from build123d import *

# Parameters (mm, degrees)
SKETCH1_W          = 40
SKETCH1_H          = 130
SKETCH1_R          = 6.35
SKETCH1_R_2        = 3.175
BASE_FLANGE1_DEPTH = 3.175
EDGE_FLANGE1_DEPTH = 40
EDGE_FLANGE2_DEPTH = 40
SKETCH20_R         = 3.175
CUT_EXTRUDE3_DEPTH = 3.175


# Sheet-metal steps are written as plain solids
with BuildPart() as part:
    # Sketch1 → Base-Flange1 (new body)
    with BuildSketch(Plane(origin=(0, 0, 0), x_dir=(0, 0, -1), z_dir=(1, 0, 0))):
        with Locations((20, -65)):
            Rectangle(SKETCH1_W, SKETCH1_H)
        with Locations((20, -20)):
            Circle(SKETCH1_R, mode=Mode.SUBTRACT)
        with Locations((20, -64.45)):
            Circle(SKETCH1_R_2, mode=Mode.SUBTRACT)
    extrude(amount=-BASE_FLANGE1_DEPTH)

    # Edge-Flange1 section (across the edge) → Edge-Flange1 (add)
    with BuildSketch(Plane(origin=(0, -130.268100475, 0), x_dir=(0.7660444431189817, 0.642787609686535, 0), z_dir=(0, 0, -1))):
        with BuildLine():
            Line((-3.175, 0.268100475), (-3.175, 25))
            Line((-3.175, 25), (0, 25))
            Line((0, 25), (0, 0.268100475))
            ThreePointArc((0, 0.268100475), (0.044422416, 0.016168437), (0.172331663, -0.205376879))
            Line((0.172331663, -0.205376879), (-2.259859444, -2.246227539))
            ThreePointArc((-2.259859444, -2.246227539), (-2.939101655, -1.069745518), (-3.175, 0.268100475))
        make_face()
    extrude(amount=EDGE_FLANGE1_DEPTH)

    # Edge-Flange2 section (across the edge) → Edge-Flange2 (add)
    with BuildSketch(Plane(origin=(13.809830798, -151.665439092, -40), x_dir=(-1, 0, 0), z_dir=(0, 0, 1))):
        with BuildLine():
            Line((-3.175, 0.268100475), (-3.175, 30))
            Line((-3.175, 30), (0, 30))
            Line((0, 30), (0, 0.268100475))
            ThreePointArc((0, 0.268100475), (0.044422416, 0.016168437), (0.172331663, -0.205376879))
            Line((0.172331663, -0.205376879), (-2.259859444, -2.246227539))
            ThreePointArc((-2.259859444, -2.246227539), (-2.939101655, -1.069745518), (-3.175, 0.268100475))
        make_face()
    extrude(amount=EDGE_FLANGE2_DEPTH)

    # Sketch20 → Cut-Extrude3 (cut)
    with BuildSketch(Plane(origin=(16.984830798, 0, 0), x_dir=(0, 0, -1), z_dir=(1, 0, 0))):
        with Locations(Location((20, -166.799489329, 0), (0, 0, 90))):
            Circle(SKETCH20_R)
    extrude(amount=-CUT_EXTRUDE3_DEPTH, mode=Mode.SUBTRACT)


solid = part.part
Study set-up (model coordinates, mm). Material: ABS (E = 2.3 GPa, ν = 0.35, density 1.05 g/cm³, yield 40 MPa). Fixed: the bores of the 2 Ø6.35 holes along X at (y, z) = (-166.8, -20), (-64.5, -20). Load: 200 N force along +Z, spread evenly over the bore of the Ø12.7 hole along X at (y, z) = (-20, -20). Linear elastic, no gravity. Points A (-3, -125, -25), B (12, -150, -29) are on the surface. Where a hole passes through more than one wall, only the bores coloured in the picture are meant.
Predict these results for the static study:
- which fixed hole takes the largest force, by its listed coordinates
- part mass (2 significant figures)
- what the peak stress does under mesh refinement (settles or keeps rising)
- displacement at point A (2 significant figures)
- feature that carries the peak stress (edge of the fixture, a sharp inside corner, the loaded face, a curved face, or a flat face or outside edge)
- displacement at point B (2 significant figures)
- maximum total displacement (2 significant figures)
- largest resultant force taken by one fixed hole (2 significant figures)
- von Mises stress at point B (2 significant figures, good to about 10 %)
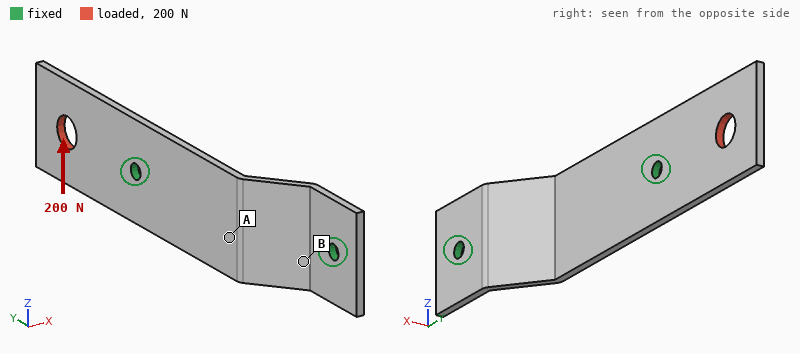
(-64.5, -20)
24 g
keeps rising
0.62 mm
edge of the fixture
0.29 mm
1.2 mm
250 N
5.6 MPa
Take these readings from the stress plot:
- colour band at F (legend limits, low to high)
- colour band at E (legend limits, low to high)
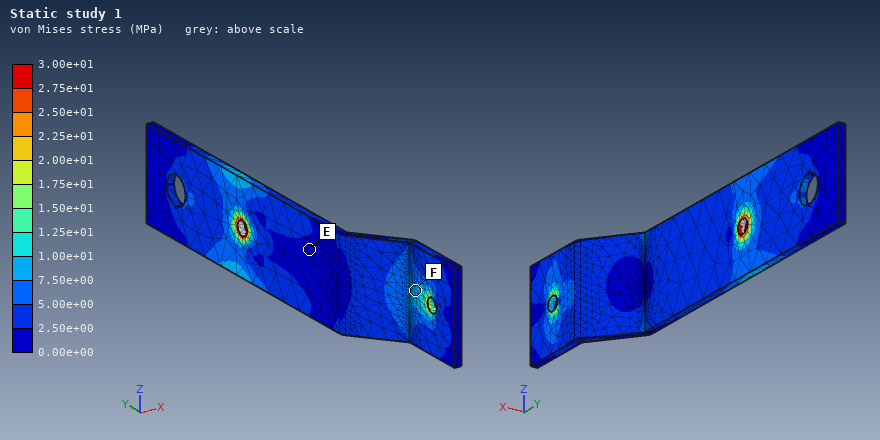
7.50e+00 to 1.00e+01 MPa
0.00e+00 to 2.50e+00 MPa
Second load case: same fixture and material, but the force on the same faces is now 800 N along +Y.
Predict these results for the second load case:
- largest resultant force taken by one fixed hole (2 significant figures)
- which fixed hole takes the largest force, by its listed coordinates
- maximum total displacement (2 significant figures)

800 N
(-64.5, -20)
0.22 mm
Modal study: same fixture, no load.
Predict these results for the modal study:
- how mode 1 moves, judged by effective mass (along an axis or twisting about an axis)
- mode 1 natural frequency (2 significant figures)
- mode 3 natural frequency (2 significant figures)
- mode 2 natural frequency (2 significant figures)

along X
190 Hz
630 Hz
550 Hz
